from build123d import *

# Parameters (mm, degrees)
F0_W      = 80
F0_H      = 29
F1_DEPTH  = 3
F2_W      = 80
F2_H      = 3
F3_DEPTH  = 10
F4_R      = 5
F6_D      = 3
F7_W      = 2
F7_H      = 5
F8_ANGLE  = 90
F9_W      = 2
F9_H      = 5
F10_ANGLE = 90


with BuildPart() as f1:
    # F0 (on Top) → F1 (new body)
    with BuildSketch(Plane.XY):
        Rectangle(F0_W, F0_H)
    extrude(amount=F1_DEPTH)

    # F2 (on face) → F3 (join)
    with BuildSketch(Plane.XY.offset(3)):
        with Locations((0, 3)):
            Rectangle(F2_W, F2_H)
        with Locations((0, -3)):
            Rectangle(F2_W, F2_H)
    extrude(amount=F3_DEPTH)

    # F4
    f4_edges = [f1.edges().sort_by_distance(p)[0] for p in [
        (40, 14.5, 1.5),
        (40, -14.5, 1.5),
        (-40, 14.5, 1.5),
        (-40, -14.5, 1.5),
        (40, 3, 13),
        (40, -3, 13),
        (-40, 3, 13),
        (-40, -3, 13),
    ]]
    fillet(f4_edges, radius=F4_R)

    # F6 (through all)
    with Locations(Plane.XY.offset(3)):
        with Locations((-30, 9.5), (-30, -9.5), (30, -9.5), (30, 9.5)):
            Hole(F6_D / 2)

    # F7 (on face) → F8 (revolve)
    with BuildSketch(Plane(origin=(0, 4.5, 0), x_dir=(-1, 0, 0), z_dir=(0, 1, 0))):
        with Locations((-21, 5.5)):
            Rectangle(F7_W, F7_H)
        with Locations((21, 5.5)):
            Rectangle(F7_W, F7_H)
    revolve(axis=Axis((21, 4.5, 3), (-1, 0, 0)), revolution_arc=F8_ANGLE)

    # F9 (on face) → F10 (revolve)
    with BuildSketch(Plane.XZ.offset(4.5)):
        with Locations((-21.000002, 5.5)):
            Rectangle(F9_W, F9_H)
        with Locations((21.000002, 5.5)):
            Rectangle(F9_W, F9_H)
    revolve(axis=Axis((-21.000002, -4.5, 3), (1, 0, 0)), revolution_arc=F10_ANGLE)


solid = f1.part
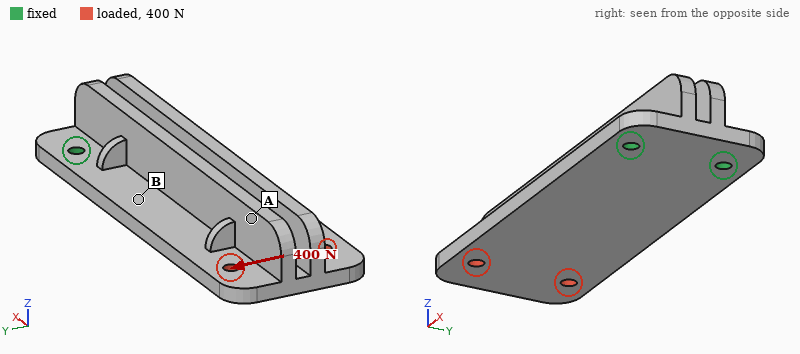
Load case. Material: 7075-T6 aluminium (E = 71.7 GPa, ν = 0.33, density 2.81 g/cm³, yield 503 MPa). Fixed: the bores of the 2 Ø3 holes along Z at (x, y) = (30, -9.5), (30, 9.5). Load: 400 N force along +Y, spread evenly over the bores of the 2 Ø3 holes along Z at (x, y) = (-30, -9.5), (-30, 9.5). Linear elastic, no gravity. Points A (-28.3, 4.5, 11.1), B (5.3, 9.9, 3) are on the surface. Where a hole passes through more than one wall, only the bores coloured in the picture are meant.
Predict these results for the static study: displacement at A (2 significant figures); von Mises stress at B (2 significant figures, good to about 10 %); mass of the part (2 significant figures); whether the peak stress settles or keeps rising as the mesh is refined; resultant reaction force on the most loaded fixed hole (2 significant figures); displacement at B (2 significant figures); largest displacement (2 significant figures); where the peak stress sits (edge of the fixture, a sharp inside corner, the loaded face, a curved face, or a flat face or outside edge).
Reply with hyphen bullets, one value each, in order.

- 72 µm
- 21 MPa
- 33 g
- keeps rising
- 1.2 kN
- 23 µm
- 96 µm
- edge of the fixture
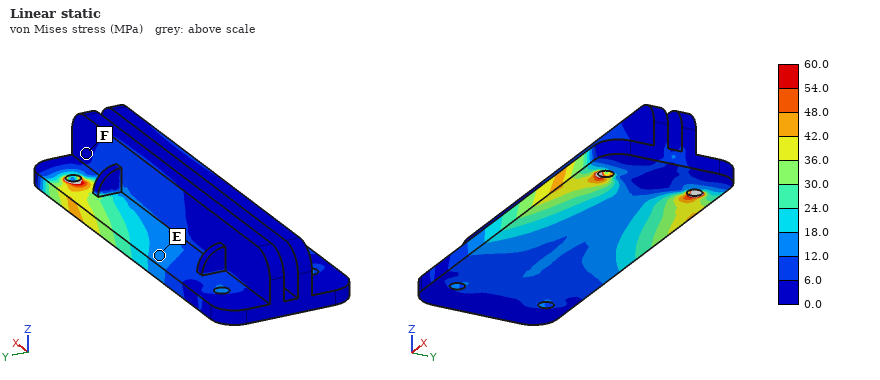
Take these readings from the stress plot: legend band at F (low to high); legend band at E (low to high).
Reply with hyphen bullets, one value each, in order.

- 0.0 to 6.0 MPa
- 12.0 to 18.0 MPa
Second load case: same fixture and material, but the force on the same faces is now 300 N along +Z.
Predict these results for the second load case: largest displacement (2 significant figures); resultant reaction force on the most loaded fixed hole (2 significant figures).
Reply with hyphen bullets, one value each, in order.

- 0.89 mm
- 220 N
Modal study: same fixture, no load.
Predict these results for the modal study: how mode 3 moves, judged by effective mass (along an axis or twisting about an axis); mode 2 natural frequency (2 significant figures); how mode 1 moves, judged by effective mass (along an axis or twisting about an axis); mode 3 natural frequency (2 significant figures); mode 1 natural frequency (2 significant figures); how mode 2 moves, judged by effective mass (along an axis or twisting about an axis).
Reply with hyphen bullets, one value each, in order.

- along Y
- 2600 Hz
- along Z
- 3700 Hz
- 900 Hz
- along Y
